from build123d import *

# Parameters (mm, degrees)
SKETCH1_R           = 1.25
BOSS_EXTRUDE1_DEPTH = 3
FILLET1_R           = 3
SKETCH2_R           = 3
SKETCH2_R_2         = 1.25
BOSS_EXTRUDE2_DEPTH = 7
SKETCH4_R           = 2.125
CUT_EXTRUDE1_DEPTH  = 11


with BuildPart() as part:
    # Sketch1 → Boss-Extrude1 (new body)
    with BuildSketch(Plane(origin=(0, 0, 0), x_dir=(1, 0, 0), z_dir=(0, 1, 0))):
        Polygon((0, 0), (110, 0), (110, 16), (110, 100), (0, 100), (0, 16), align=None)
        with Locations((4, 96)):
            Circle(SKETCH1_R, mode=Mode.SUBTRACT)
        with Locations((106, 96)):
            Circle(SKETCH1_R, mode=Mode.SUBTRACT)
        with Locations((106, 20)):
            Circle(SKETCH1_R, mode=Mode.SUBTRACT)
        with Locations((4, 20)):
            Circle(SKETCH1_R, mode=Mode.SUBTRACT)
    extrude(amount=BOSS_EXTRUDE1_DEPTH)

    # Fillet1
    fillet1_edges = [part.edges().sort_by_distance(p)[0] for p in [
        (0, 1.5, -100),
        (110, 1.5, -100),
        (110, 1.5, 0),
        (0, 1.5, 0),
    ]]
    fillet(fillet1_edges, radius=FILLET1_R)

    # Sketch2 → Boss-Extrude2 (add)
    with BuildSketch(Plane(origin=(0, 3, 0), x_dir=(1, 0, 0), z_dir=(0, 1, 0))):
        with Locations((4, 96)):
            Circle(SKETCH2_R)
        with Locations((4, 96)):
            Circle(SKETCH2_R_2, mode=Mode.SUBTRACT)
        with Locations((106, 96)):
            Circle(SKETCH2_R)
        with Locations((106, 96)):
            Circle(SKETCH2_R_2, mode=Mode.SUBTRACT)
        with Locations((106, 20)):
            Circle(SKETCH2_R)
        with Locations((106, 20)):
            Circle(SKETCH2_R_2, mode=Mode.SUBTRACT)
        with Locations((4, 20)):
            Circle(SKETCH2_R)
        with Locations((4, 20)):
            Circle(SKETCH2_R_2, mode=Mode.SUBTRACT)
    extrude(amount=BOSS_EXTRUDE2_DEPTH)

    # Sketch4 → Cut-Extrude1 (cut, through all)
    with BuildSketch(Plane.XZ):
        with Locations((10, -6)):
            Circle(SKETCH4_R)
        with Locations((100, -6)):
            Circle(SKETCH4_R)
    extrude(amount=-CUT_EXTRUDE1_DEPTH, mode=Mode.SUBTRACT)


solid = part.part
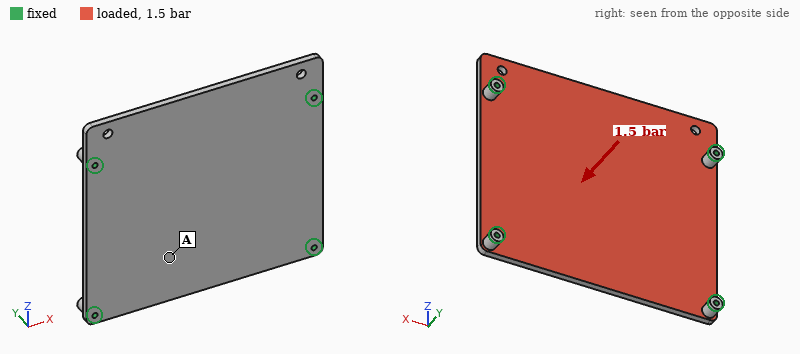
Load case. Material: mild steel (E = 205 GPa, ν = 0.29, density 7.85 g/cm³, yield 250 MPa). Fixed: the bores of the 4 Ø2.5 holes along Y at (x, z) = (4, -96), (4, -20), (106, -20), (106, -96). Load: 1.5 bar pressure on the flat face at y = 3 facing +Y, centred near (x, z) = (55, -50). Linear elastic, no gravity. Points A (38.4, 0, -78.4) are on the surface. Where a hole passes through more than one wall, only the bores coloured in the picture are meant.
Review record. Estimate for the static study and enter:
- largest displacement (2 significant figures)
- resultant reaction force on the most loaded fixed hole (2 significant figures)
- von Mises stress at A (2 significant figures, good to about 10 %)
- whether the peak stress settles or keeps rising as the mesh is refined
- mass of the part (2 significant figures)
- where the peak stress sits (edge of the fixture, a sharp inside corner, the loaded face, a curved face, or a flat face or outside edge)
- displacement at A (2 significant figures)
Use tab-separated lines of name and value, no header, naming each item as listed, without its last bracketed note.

largest displacement	0.17 mm
resultant reaction force on the most loaded fixed hole	500 N
von Mises stress at A	42 MPa
whether the peak stress settles or keeps rising as the mesh is refined	keeps rising
mass of the part	260 g
where the peak stress sits	edge of the fixture
displacement at A	0.14 mm
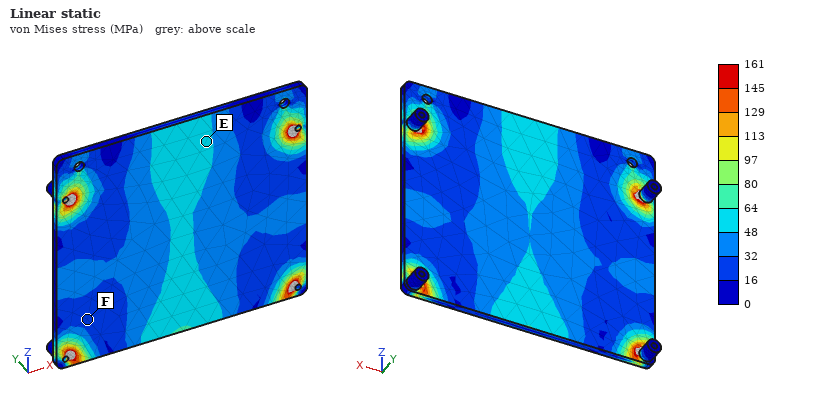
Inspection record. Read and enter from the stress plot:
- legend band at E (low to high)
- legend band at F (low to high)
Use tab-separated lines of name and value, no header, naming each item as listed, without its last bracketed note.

legend band at E	48 to 64 MPa
legend band at F	16 to 32 MPa
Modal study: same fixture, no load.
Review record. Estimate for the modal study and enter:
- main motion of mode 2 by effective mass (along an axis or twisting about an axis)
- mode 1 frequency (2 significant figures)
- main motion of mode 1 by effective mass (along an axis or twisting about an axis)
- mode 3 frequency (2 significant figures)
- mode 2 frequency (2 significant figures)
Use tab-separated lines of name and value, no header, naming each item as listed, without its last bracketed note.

main motion of mode 2 by effective mass	twisting about X
mode 1 frequency	1100 Hz
main motion of mode 1 by effective mass	along Y
mode 3 frequency	2400 Hz
mode 2 frequency	1600 Hz
